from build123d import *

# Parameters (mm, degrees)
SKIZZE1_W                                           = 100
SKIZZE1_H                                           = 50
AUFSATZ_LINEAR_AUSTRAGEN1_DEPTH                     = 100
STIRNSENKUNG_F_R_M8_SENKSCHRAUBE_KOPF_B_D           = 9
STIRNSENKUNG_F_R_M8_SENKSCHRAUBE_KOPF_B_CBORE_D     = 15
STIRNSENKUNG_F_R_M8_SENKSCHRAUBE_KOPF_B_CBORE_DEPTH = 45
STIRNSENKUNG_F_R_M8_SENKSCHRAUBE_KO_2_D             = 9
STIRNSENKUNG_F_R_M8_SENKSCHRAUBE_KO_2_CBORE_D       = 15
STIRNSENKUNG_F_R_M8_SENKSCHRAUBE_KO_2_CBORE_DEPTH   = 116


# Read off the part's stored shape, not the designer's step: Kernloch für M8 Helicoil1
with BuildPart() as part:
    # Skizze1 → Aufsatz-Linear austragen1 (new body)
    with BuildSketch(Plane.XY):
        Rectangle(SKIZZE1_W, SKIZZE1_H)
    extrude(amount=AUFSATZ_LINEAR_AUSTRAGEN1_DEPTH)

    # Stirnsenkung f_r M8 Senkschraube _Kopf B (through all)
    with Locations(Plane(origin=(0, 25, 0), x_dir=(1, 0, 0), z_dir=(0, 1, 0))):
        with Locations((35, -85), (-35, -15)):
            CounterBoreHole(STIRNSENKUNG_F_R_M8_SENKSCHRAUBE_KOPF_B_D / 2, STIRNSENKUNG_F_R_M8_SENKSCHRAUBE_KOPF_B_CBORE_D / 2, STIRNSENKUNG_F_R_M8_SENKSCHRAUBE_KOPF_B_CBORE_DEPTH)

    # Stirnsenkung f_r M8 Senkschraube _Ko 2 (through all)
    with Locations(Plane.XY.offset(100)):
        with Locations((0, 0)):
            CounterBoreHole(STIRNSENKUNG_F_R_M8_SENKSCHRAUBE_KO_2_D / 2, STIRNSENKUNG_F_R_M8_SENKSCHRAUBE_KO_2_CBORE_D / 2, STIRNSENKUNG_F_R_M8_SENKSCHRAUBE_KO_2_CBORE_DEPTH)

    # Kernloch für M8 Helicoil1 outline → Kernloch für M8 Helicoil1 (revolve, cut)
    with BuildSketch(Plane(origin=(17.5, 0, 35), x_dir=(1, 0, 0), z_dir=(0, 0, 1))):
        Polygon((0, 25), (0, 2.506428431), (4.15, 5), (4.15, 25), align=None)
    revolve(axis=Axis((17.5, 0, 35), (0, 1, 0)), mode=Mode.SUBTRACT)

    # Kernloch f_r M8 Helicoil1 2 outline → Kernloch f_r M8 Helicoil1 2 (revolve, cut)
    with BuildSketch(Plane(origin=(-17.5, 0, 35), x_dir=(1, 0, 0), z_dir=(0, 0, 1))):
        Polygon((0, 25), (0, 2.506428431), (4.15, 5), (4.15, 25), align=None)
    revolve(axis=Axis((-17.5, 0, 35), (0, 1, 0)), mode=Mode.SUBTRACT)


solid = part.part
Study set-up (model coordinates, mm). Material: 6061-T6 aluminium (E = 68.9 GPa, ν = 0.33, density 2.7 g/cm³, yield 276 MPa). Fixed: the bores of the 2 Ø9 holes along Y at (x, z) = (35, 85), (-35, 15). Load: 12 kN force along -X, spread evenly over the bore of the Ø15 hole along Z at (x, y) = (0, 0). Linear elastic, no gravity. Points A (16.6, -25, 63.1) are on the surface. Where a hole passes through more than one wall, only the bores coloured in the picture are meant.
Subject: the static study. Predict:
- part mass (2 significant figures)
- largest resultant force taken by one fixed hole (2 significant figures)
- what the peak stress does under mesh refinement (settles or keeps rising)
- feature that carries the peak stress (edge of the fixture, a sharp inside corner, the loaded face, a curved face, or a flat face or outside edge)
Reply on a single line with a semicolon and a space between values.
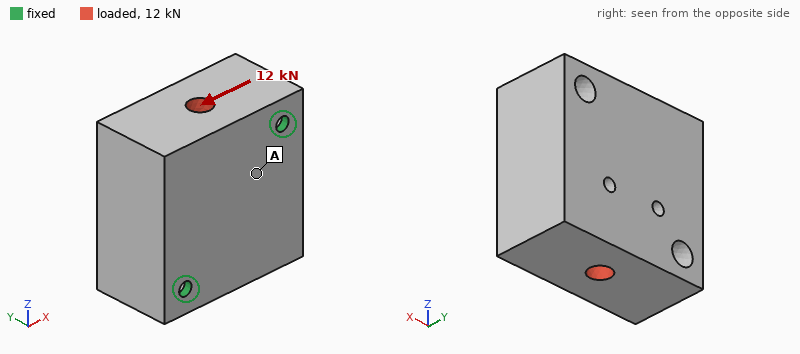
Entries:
1.3 kg; 6.3 kN; keeps rising; edge of the fixture
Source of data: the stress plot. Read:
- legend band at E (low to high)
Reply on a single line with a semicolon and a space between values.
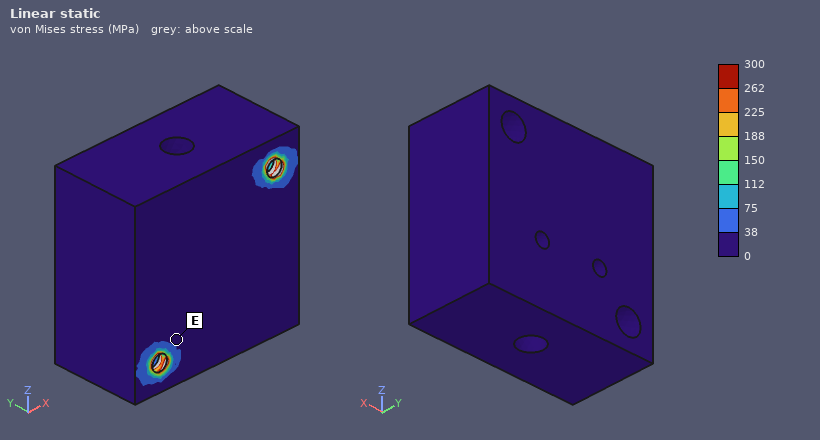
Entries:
0 to 38 MPa
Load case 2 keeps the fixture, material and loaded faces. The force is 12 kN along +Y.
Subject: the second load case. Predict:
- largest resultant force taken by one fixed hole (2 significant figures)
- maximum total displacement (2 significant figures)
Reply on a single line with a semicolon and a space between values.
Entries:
6.4 kN; 17 µm
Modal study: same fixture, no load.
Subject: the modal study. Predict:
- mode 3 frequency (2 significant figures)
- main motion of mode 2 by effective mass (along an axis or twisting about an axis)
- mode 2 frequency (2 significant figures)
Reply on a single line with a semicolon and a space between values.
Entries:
4700 Hz; along Y; 4100 Hz
